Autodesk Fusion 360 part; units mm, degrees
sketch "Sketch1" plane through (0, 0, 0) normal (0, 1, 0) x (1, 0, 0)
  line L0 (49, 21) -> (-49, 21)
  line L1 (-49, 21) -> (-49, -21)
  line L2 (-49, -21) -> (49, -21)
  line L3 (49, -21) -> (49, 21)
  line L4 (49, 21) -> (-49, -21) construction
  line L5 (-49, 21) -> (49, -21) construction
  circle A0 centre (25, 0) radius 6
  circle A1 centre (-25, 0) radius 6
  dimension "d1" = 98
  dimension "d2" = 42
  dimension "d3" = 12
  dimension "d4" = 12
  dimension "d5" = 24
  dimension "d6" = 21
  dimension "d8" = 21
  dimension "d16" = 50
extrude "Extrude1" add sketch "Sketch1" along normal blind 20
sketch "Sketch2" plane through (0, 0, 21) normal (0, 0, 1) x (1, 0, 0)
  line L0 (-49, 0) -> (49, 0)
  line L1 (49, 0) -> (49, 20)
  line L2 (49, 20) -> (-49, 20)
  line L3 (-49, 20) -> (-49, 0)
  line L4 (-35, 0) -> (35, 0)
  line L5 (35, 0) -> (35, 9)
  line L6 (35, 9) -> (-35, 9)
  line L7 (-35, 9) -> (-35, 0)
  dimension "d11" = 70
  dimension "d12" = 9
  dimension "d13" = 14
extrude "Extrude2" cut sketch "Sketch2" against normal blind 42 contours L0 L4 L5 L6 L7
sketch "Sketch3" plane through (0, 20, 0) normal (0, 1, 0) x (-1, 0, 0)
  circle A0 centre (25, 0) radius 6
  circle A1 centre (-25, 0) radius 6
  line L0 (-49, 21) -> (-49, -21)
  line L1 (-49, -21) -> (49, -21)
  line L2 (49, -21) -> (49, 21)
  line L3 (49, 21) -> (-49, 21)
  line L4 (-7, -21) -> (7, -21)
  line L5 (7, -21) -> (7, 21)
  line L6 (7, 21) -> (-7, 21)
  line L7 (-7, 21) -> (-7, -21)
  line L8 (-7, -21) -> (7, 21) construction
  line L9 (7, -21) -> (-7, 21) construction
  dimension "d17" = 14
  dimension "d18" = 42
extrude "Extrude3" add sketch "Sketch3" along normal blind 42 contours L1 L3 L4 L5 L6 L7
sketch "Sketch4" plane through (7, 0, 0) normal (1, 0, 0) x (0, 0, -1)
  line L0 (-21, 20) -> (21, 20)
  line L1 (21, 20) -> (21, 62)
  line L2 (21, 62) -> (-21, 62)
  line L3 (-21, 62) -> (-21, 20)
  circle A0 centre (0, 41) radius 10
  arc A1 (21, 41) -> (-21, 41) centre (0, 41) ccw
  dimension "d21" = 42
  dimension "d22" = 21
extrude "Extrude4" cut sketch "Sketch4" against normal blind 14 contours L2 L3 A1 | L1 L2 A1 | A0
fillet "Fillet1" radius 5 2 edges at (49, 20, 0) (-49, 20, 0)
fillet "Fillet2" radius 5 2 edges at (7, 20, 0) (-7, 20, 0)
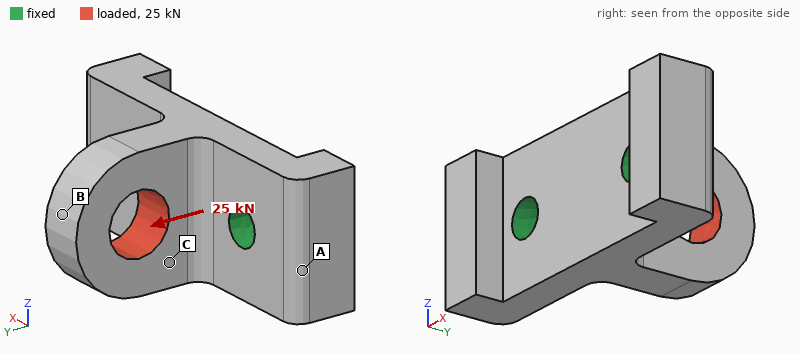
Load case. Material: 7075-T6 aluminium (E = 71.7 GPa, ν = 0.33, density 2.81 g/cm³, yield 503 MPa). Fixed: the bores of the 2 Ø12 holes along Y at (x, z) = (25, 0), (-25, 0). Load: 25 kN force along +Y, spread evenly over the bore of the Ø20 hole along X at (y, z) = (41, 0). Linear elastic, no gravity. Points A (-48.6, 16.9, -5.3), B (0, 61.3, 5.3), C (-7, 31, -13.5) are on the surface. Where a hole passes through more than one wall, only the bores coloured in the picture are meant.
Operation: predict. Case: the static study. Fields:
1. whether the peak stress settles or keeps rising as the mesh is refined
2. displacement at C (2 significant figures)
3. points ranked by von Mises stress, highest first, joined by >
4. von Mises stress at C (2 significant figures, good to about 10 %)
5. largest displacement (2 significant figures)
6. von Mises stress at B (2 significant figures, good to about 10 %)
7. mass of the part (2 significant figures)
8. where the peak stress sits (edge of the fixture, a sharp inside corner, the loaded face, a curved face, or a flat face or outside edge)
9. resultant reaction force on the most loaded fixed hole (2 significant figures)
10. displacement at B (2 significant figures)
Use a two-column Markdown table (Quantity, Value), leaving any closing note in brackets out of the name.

| Quantity | Value |
|---|---|
| whether the peak stress settles or keeps rising as the mesh is refined | keeps rising |
| displacement at C | 53 µm |
| points ranked by von Mises stress, highest first, joined by > | C > B > A |
| von Mises stress at C | 65 MPa |
| largest displacement | 84 µm |
| von Mises stress at B | 49 MPa |
| mass of the part | 200 g |
| where the peak stress sits | edge of the fixture |
| resultant reaction force on the most loaded fixed hole | 13 kN |
| displacement at B | 77 µm |
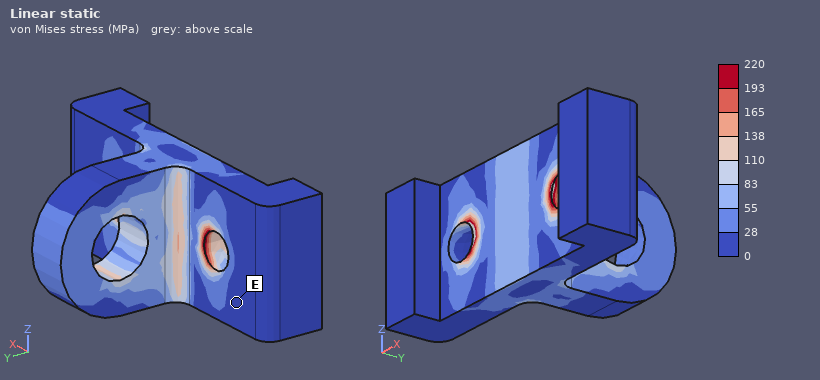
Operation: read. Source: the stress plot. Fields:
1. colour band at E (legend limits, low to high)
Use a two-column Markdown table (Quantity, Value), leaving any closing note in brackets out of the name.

| Quantity | Value |
|---|---|
| colour band at E | 0 to 28 MPa |
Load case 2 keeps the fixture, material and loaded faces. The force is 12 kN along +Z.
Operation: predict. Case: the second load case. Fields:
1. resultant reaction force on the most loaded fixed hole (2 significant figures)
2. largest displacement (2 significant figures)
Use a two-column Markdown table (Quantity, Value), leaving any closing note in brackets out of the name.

| Quantity | Value |
|---|---|
| resultant reaction force on the most loaded fixed hole | 6.0 kN |
| largest displacement | 0.28 mm |
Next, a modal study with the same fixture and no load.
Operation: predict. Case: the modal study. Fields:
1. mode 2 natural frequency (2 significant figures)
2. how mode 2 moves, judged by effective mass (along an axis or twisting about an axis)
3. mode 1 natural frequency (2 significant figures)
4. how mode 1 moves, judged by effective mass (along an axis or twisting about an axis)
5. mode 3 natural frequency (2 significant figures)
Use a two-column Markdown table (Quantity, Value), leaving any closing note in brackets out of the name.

| Quantity | Value |
|---|---|
| mode 2 natural frequency | 5800 Hz |
| how mode 2 moves, judged by effective mass | along X |
| mode 1 natural frequency | 5400 Hz |
| how mode 1 moves, judged by effective mass | along Z |
| mode 3 natural frequency | 11 kHz |
